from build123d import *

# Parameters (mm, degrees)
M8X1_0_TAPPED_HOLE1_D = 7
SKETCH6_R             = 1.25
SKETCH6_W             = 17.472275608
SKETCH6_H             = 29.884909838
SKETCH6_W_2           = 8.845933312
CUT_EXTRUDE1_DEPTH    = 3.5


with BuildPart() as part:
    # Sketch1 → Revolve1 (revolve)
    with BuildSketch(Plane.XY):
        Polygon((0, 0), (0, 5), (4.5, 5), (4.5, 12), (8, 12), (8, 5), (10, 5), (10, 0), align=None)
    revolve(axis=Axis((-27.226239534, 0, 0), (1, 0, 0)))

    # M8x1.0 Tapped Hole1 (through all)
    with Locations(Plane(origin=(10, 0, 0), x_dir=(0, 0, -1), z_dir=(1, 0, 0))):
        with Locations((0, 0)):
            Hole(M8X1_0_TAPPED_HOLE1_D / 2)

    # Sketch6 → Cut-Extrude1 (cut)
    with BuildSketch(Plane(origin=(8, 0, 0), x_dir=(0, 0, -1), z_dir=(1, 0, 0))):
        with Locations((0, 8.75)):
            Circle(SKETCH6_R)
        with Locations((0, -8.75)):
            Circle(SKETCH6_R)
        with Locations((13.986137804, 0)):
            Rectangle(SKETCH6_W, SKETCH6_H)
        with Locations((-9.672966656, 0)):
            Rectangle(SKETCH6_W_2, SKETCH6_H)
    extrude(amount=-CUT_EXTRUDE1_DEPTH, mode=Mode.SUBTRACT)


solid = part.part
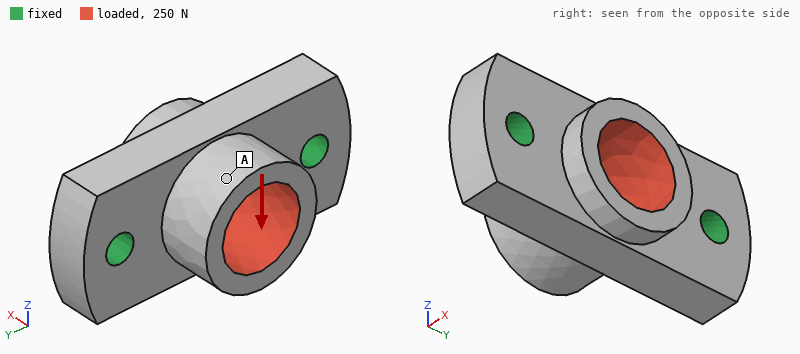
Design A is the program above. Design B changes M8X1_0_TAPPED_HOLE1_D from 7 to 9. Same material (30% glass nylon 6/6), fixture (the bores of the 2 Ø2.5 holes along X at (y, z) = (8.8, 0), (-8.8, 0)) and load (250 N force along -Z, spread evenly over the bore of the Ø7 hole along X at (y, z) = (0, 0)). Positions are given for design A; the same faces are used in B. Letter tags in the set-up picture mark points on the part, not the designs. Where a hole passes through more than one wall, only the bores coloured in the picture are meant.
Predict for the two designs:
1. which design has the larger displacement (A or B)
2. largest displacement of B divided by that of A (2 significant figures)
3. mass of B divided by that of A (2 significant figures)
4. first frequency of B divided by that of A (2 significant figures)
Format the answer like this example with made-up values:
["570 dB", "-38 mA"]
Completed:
["B", "1.7", "0.73", "1.2"]
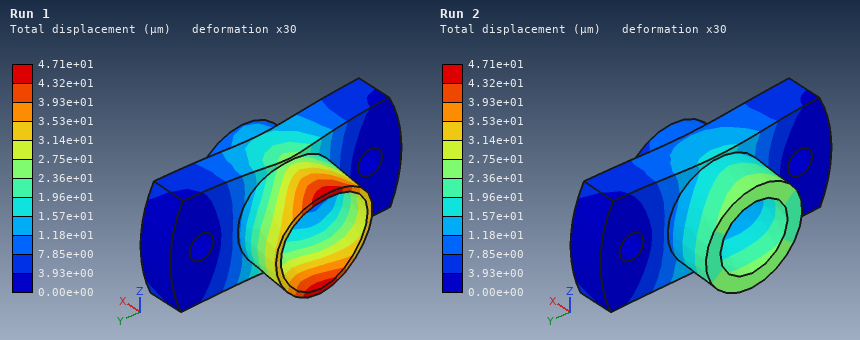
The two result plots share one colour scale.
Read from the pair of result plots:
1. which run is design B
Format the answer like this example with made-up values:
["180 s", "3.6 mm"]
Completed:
["Run 1"]
